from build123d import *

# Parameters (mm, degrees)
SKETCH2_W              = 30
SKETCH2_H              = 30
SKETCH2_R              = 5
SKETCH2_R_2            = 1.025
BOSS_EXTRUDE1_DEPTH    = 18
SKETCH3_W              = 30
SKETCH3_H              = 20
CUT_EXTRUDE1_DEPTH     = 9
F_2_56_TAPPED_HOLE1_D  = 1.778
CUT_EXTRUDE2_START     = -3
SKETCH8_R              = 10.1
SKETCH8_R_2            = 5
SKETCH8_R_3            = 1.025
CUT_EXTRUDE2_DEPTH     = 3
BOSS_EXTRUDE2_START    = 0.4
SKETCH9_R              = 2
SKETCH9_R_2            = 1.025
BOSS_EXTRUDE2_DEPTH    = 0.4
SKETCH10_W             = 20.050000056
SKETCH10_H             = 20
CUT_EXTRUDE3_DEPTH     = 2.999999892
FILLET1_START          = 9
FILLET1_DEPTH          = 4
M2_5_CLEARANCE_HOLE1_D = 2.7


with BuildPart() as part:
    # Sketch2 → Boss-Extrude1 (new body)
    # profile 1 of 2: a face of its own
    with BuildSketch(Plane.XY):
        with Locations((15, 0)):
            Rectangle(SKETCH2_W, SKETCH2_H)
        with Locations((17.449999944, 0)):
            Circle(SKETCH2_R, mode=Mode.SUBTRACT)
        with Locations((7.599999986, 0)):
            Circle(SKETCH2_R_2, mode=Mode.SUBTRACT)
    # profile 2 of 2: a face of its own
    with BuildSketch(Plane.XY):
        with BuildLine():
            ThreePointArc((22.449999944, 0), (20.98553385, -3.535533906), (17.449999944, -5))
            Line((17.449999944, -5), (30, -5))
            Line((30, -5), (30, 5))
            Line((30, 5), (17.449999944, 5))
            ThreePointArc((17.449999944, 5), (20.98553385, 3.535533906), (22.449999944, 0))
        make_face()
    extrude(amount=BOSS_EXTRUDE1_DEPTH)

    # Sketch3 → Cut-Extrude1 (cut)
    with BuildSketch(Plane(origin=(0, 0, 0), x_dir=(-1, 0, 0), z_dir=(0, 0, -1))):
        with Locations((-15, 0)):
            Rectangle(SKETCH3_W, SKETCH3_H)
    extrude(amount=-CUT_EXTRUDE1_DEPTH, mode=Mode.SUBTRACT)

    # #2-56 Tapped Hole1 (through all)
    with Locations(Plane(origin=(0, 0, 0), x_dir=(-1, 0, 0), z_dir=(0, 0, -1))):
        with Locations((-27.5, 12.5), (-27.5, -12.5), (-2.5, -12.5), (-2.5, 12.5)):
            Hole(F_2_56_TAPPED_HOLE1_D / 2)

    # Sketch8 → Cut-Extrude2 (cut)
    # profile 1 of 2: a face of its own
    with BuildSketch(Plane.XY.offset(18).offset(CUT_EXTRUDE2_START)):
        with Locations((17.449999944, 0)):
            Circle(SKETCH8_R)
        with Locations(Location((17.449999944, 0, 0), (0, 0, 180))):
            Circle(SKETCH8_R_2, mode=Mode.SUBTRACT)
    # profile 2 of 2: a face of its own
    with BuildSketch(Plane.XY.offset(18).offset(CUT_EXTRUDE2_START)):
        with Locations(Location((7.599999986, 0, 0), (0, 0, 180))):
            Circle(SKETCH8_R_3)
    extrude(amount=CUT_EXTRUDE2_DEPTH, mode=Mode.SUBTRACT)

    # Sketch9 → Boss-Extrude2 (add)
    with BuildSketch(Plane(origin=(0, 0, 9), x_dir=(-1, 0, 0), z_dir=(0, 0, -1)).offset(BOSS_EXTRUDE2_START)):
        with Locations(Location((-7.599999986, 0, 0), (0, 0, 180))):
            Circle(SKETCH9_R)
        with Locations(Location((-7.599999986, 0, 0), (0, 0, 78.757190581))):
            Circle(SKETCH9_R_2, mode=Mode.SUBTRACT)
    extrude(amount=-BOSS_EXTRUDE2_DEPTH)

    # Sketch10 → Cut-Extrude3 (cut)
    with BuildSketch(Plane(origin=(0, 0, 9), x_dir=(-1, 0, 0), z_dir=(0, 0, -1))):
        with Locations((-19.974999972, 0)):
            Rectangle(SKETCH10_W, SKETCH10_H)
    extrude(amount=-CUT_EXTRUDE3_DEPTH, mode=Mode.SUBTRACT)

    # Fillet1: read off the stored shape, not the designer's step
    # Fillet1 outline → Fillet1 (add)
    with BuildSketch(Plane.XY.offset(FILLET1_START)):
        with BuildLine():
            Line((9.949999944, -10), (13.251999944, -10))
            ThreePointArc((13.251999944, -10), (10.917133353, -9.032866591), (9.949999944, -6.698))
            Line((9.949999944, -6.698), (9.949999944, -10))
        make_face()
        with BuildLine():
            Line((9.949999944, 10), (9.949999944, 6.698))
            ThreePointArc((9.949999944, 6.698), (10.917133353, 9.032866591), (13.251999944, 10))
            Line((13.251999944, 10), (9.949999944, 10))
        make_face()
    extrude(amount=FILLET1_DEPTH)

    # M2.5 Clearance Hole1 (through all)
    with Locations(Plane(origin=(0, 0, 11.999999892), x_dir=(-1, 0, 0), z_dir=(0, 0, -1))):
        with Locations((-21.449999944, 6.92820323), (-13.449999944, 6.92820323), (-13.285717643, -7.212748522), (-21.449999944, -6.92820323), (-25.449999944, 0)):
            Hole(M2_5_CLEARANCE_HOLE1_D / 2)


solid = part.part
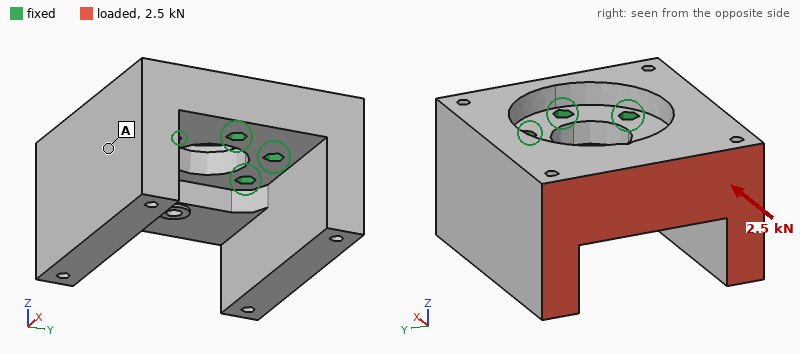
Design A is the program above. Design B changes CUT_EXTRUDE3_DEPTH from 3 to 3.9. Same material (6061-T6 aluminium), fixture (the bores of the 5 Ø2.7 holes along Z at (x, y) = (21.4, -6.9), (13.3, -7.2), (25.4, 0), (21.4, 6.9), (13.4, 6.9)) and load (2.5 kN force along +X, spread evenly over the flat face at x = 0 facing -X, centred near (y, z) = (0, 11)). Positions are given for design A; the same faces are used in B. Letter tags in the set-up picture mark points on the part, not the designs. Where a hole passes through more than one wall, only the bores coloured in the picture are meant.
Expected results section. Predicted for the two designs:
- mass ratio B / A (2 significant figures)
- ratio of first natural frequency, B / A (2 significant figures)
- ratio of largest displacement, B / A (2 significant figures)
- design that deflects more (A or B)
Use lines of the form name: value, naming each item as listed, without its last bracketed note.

mass ratio B / A: 0.97
ratio of first natural frequency, B / A: 0.81
ratio of largest displacement, B / A: 1.6
design that deflects more: B
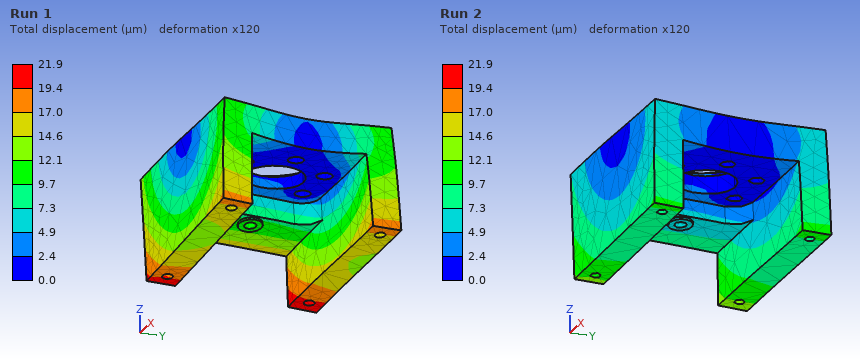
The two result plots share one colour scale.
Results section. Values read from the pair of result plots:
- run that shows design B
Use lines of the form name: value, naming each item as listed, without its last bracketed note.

run that shows design B: Run 1
